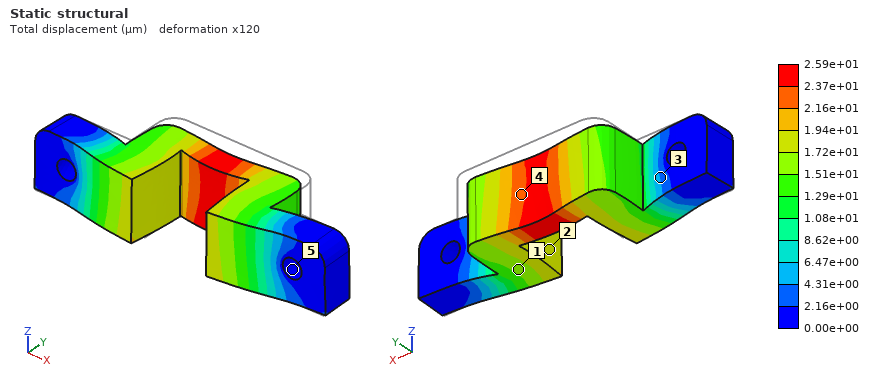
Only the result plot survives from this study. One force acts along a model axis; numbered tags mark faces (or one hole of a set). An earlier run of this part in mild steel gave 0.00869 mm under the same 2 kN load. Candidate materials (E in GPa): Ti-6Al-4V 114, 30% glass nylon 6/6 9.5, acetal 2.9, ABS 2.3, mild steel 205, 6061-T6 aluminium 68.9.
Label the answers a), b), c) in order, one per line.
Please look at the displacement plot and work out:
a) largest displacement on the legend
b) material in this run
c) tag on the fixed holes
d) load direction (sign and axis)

a) 2.59e+01 µm
b) 6061-T6 aluminium
c) 5
d) -Y
